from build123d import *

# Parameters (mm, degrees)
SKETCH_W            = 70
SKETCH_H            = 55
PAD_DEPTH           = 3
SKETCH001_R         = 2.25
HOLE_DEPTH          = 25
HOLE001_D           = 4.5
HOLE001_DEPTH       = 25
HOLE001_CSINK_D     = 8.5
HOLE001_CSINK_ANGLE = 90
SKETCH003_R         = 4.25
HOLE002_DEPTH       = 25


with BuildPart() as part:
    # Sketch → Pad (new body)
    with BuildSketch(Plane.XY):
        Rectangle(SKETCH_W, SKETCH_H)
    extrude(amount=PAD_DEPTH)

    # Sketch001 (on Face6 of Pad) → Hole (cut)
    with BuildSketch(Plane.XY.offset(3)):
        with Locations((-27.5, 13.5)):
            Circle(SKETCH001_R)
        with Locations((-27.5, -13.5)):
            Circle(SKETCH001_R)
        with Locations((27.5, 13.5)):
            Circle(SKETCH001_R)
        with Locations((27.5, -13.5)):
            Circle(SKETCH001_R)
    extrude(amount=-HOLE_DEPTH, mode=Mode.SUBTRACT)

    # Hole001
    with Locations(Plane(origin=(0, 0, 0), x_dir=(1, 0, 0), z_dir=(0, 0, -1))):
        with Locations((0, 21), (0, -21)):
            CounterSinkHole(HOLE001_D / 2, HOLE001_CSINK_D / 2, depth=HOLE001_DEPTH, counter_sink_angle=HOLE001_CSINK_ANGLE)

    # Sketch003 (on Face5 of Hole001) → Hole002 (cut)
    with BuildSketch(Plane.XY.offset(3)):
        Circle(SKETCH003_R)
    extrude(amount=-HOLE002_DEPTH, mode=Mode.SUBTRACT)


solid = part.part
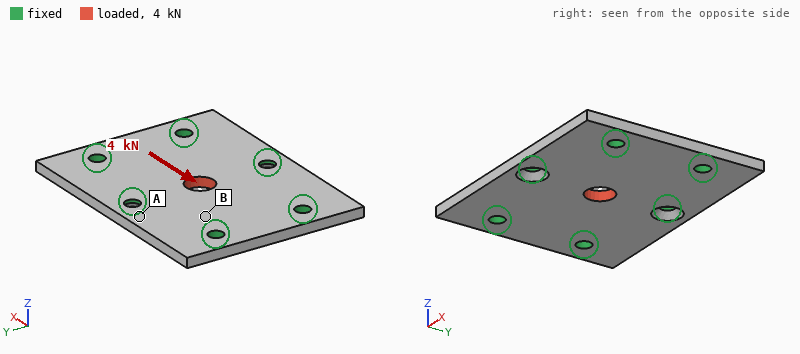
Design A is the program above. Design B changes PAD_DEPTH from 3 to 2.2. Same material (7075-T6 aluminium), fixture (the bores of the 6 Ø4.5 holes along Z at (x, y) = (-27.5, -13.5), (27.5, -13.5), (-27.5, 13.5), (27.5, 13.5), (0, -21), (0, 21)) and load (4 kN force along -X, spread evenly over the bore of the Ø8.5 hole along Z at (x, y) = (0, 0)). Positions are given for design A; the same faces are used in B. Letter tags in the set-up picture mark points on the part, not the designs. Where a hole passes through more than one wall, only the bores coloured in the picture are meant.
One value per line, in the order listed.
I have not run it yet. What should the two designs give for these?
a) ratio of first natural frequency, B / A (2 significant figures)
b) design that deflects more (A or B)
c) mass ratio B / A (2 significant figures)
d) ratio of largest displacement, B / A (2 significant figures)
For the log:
0.74
B
0.73
1.4
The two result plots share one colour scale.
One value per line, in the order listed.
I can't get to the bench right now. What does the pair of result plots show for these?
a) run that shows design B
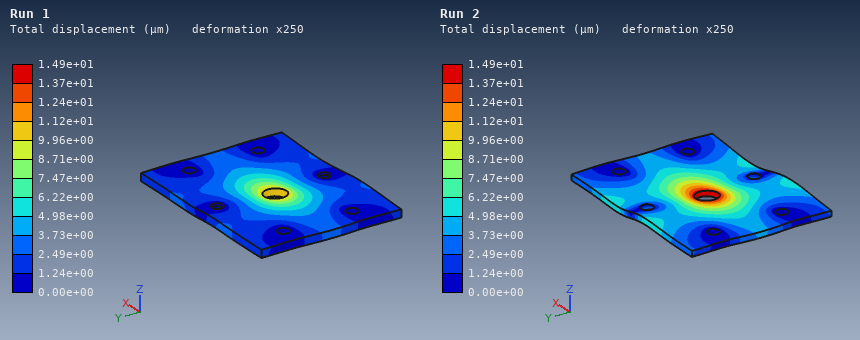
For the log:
Run 2
